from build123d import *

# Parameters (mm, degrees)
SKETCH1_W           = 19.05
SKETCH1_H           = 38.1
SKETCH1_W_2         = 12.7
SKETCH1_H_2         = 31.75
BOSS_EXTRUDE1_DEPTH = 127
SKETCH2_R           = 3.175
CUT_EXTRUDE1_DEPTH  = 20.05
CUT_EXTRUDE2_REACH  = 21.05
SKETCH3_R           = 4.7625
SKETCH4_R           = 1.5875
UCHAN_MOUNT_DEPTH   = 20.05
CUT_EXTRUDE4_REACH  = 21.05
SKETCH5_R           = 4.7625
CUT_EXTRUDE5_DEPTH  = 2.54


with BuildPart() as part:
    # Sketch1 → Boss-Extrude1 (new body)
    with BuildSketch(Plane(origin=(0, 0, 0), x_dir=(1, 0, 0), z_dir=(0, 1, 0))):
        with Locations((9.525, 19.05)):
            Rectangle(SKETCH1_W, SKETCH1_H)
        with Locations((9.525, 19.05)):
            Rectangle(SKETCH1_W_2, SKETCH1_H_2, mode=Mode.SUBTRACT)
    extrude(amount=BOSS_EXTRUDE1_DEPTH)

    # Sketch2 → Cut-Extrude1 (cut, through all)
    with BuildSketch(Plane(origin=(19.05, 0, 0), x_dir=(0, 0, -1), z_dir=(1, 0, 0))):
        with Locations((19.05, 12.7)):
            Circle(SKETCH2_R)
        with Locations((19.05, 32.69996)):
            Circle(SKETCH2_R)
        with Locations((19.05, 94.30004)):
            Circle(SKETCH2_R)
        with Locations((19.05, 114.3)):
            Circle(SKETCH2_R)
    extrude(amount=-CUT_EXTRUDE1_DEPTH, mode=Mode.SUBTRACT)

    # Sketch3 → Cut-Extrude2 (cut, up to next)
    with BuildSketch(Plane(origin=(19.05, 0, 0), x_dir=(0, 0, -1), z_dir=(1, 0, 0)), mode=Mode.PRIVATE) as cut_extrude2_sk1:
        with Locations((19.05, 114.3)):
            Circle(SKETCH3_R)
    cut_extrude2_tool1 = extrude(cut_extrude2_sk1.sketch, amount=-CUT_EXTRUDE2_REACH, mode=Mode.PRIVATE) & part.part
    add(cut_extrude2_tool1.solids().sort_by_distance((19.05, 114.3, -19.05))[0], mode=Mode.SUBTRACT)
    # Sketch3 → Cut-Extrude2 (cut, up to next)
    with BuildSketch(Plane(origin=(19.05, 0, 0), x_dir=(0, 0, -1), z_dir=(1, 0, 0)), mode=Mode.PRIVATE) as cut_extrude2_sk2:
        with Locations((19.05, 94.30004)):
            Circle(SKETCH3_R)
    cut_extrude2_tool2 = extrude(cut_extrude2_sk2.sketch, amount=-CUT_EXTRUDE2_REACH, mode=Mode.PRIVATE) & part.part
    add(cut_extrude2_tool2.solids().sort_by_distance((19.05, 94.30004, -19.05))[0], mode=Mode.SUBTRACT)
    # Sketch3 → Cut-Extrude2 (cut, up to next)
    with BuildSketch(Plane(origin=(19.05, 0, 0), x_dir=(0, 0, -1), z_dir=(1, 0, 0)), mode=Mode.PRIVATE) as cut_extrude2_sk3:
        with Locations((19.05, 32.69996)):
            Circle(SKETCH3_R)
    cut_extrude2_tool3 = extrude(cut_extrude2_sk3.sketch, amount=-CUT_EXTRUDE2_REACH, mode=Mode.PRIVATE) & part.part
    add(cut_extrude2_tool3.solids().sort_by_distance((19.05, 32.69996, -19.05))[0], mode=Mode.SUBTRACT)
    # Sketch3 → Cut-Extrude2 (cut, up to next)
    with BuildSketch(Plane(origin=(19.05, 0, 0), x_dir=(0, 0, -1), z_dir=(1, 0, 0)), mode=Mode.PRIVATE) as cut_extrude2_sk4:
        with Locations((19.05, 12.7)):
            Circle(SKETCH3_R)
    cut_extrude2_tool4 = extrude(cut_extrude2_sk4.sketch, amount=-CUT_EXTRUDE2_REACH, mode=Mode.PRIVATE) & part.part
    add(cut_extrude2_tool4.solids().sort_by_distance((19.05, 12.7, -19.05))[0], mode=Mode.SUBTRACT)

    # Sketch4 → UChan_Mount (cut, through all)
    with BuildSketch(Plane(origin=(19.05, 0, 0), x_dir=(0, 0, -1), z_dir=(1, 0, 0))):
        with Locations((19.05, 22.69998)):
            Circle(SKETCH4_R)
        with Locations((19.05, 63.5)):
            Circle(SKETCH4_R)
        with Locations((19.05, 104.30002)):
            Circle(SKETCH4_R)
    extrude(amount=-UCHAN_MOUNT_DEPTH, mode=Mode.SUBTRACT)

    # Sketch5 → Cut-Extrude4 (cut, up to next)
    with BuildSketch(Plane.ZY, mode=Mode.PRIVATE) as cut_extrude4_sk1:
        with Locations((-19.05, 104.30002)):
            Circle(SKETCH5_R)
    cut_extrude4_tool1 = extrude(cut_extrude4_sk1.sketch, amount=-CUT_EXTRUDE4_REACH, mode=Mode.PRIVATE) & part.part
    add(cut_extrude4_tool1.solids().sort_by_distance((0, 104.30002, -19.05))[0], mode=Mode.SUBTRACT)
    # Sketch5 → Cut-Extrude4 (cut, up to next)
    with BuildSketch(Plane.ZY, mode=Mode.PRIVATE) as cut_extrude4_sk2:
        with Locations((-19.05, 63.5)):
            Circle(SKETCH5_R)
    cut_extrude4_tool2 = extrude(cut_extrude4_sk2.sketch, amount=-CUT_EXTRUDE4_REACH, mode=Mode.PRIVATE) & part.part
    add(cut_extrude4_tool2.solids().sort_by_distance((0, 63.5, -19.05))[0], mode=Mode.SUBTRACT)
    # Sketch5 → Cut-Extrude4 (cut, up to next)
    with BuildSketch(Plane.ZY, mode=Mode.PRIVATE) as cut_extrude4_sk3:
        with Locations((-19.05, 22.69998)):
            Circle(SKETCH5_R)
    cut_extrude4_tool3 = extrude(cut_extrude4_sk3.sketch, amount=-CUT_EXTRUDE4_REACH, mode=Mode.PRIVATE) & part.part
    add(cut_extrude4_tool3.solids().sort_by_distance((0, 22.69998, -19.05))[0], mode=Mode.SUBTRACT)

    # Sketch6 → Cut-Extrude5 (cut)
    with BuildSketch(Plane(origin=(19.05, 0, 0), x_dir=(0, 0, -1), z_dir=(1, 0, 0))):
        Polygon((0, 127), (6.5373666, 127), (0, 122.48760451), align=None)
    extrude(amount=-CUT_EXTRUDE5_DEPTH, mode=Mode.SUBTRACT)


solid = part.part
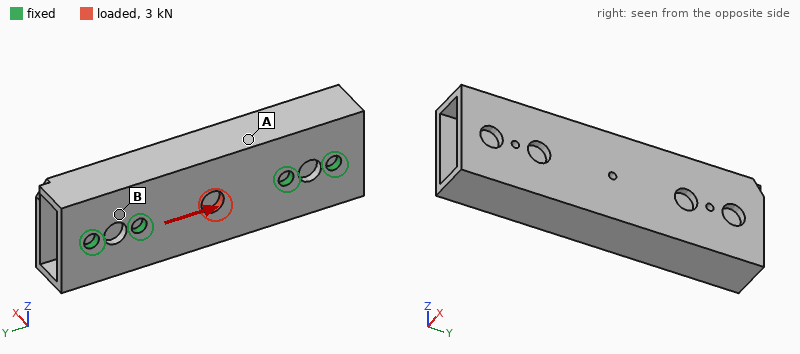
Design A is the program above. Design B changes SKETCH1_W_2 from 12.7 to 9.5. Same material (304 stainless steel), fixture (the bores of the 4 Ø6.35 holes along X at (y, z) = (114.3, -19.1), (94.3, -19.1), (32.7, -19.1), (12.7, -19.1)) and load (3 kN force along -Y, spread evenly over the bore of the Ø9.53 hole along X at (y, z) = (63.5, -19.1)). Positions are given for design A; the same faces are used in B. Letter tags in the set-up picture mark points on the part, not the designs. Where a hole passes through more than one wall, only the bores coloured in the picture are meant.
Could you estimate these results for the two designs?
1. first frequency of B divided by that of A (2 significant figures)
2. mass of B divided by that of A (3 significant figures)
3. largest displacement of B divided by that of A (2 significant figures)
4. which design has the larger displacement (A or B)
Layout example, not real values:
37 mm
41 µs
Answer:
1.6
1.31
0.67
A
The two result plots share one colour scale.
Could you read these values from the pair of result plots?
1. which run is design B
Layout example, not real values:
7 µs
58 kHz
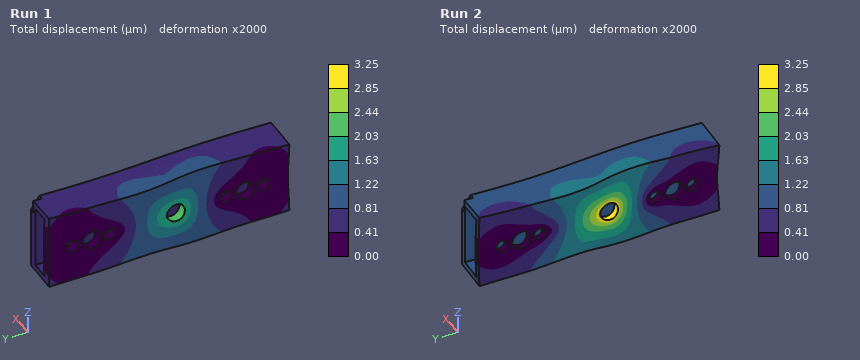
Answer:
Run 1
